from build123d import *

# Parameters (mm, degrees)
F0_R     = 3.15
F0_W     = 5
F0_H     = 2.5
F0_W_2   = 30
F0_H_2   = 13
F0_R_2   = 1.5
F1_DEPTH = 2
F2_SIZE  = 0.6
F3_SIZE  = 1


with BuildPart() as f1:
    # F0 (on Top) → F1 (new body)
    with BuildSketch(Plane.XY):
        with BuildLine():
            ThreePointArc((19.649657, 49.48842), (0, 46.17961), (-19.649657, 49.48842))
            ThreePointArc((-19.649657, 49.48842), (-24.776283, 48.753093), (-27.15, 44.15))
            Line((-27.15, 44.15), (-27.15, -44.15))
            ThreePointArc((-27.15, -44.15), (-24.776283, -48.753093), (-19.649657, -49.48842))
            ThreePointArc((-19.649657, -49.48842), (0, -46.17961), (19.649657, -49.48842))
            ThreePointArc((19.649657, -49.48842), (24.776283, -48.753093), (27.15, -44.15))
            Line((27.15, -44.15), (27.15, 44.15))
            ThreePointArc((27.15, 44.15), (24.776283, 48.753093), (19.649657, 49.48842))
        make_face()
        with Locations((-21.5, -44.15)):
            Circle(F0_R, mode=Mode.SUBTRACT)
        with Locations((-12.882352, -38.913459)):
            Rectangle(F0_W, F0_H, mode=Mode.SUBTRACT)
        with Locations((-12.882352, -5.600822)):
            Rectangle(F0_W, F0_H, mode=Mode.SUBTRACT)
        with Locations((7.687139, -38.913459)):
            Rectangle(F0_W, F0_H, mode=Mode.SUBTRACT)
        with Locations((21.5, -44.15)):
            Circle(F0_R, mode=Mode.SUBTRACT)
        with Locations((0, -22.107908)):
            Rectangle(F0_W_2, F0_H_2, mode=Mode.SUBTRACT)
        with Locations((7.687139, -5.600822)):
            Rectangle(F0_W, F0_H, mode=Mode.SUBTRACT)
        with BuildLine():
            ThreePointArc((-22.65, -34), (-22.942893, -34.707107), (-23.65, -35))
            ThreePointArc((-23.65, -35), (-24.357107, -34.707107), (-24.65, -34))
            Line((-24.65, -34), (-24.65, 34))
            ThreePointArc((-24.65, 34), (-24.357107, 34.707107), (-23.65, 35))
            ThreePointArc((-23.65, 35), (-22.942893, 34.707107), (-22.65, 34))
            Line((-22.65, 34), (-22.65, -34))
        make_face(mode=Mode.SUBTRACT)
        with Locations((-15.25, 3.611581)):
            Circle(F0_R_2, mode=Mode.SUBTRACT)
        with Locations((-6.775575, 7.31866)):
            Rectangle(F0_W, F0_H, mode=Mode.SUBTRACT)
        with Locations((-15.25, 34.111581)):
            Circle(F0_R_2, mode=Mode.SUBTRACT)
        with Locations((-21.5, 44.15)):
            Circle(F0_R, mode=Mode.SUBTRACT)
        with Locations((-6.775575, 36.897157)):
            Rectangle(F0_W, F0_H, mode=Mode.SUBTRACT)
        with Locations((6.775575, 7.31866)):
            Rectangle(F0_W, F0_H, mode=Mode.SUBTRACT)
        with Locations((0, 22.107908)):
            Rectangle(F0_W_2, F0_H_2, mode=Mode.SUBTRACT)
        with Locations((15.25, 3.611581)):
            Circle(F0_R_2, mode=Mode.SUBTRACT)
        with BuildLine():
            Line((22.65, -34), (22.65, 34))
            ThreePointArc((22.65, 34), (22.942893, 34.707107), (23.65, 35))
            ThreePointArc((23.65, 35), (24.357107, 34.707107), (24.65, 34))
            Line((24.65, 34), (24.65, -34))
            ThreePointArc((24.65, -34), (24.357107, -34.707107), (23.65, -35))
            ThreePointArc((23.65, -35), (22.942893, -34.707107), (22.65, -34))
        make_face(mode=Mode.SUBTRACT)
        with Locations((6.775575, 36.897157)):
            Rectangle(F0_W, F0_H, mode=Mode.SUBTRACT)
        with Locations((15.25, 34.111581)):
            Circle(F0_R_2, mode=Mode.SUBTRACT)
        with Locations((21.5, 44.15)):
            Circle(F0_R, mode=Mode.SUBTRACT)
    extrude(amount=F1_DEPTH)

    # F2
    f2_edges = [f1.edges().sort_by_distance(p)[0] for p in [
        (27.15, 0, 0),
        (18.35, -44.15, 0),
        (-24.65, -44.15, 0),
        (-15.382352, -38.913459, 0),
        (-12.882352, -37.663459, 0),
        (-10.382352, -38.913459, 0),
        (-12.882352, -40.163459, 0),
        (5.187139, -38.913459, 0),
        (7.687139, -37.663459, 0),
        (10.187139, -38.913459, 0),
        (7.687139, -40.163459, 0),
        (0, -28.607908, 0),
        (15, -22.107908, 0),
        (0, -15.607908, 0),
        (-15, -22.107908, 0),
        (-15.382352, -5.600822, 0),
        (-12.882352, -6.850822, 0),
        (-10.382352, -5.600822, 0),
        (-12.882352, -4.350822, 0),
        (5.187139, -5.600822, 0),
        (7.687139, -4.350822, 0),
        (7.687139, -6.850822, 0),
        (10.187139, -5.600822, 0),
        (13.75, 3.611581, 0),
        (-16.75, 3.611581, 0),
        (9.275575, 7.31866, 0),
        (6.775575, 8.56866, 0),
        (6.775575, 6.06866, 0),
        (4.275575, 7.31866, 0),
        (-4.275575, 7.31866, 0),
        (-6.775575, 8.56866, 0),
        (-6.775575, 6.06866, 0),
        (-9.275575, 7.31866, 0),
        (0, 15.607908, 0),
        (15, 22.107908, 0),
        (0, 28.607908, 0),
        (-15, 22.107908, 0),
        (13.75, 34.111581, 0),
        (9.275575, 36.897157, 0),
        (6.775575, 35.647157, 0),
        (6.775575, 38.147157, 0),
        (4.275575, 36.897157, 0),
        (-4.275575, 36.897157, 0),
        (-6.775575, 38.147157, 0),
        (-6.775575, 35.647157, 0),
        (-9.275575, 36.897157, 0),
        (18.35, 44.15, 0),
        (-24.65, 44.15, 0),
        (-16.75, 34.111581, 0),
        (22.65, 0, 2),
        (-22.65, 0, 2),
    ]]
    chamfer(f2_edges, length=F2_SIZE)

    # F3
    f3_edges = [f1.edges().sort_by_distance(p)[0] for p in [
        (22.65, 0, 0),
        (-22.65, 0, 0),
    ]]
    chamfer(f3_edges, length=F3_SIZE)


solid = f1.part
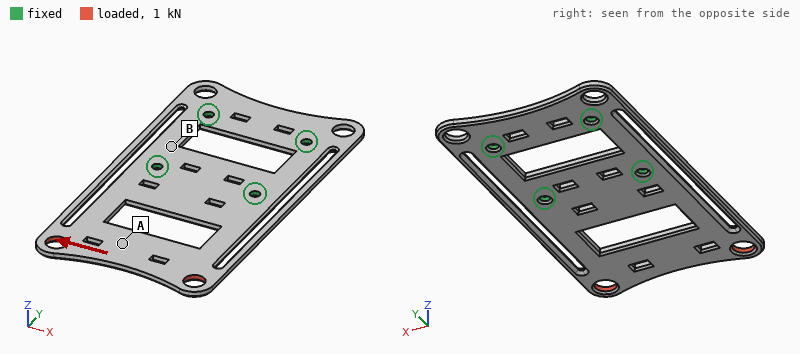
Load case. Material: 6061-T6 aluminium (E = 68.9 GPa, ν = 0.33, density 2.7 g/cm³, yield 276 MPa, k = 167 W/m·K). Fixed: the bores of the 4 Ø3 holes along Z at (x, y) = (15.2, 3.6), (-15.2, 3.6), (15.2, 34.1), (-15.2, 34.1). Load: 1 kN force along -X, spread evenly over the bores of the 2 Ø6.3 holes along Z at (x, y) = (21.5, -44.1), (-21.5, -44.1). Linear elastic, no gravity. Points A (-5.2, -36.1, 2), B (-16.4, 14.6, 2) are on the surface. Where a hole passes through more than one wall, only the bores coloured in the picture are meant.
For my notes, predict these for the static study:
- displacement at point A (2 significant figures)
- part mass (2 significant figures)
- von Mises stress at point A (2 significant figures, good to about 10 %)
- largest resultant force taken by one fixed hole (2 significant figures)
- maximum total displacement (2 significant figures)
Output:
0.18 mm
20 g
44 MPa
1.3 kN
0.26 mm
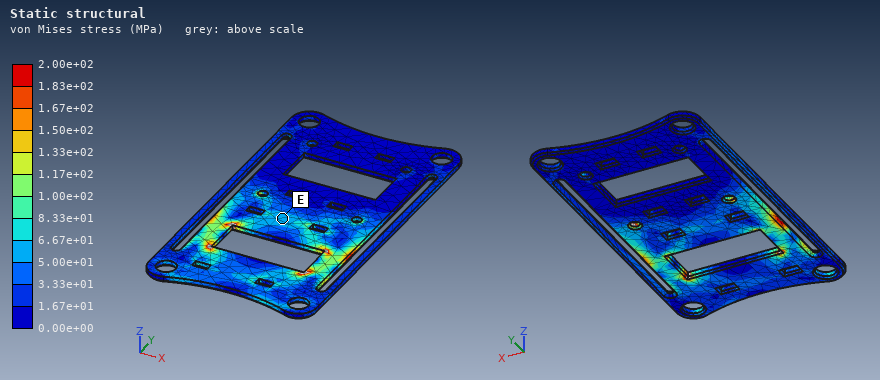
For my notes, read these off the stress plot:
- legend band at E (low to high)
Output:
5.00e+01 to 6.67e+01 MPa
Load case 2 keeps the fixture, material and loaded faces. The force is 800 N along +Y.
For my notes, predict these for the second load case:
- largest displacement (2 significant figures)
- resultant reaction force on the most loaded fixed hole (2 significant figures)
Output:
0.27 mm
340 N
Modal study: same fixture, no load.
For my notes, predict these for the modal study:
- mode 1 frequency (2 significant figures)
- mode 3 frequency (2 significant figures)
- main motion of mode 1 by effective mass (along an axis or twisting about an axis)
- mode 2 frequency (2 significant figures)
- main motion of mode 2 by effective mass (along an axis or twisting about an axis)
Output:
490 Hz
1500 Hz
along Z
1100 Hz
twisting about Y
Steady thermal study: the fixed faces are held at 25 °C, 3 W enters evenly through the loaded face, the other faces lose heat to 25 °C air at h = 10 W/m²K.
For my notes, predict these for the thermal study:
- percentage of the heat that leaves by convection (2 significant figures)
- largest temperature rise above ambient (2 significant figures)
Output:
16 %
19 K
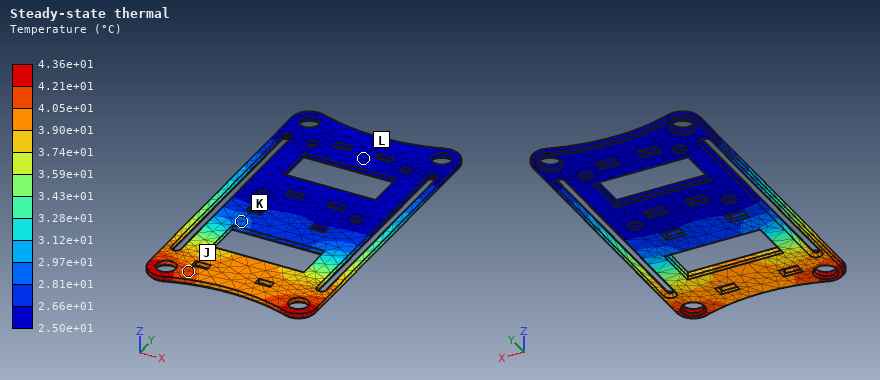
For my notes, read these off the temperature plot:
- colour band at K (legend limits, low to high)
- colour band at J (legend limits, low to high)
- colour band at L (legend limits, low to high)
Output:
2.81e+01 to 2.97e+01 °C
4.05e+01 to 4.21e+01 °C
2.50e+01 to 2.66e+01 °C
